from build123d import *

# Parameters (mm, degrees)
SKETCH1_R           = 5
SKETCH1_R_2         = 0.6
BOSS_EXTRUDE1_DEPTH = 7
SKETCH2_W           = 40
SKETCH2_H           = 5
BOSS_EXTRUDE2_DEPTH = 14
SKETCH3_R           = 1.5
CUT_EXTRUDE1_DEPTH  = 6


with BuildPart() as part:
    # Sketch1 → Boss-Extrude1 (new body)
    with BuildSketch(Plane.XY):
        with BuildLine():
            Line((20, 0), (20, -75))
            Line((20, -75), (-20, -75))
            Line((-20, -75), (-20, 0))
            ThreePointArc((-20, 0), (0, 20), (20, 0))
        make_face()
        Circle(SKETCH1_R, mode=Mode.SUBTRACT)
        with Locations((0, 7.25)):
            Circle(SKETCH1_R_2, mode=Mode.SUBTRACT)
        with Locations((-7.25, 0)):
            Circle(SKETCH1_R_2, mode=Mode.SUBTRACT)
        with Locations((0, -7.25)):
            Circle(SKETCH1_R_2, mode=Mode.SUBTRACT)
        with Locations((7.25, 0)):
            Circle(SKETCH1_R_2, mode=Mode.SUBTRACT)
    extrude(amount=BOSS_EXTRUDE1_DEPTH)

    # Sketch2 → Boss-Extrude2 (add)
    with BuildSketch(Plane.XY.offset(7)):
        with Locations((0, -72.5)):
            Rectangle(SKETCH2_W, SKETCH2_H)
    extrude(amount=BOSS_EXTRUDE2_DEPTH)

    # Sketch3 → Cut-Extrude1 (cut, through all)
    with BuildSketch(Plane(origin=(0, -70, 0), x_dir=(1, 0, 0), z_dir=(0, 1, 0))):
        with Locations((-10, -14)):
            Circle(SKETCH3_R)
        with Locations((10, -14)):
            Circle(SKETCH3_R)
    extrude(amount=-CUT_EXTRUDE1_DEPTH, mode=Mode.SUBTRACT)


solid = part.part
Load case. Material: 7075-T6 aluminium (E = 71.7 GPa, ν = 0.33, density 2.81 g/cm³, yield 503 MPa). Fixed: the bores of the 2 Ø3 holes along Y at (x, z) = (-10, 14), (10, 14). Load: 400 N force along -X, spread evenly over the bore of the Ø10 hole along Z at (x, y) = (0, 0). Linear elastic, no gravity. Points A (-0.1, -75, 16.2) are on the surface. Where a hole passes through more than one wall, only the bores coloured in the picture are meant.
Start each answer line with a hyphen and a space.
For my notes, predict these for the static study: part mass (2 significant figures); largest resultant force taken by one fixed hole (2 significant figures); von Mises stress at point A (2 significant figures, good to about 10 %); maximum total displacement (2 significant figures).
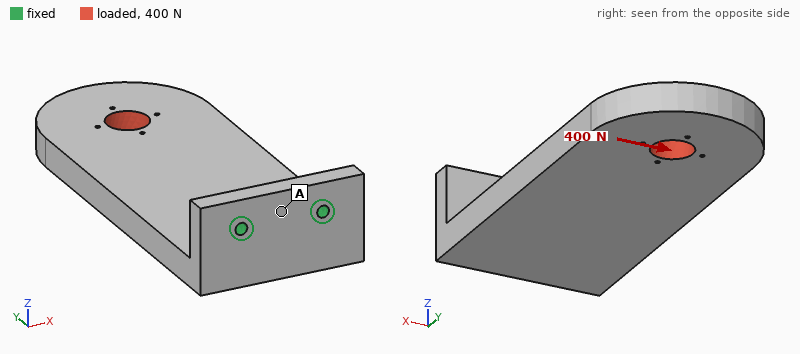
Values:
- 77 g
- 1.2 kN
- 16 MPa
- 0.19 mm
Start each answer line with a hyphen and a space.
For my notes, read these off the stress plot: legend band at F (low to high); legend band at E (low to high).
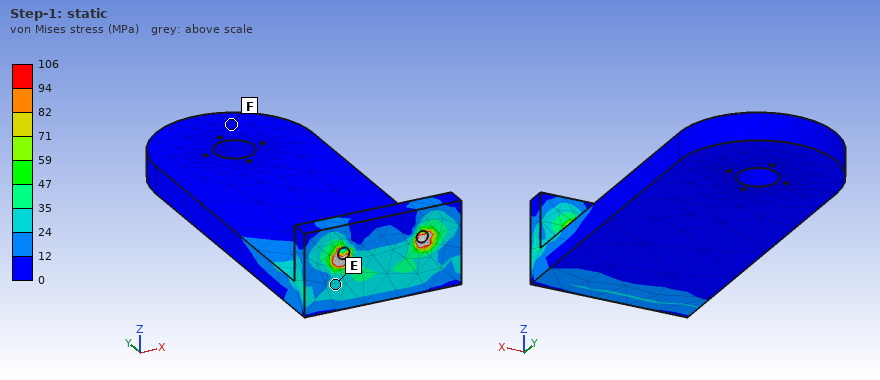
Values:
- 0 to 12 MPa
- 24 to 35 MPa
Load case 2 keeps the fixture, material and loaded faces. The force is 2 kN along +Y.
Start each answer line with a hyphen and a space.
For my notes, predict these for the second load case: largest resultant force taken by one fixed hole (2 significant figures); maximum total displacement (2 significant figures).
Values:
- 1.0 kN
- 0.44 mm
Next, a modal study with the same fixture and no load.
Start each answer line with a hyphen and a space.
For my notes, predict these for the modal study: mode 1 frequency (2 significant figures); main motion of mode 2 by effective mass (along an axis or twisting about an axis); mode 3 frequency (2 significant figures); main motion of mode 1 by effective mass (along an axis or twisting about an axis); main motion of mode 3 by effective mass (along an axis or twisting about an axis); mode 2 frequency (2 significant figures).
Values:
- 500 Hz
- along X
- 3200 Hz
- along Z
- twisting about Y
- 1400 Hz
